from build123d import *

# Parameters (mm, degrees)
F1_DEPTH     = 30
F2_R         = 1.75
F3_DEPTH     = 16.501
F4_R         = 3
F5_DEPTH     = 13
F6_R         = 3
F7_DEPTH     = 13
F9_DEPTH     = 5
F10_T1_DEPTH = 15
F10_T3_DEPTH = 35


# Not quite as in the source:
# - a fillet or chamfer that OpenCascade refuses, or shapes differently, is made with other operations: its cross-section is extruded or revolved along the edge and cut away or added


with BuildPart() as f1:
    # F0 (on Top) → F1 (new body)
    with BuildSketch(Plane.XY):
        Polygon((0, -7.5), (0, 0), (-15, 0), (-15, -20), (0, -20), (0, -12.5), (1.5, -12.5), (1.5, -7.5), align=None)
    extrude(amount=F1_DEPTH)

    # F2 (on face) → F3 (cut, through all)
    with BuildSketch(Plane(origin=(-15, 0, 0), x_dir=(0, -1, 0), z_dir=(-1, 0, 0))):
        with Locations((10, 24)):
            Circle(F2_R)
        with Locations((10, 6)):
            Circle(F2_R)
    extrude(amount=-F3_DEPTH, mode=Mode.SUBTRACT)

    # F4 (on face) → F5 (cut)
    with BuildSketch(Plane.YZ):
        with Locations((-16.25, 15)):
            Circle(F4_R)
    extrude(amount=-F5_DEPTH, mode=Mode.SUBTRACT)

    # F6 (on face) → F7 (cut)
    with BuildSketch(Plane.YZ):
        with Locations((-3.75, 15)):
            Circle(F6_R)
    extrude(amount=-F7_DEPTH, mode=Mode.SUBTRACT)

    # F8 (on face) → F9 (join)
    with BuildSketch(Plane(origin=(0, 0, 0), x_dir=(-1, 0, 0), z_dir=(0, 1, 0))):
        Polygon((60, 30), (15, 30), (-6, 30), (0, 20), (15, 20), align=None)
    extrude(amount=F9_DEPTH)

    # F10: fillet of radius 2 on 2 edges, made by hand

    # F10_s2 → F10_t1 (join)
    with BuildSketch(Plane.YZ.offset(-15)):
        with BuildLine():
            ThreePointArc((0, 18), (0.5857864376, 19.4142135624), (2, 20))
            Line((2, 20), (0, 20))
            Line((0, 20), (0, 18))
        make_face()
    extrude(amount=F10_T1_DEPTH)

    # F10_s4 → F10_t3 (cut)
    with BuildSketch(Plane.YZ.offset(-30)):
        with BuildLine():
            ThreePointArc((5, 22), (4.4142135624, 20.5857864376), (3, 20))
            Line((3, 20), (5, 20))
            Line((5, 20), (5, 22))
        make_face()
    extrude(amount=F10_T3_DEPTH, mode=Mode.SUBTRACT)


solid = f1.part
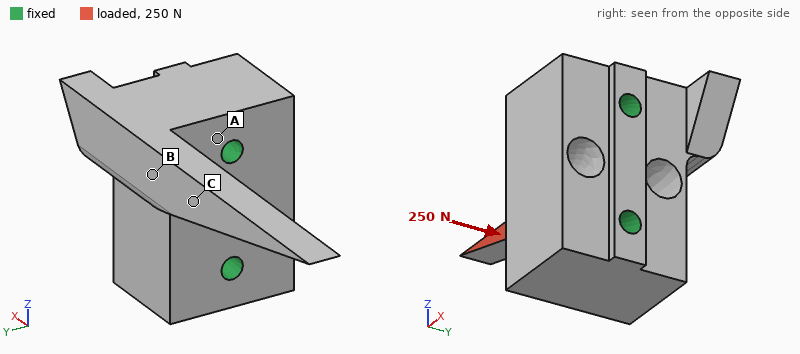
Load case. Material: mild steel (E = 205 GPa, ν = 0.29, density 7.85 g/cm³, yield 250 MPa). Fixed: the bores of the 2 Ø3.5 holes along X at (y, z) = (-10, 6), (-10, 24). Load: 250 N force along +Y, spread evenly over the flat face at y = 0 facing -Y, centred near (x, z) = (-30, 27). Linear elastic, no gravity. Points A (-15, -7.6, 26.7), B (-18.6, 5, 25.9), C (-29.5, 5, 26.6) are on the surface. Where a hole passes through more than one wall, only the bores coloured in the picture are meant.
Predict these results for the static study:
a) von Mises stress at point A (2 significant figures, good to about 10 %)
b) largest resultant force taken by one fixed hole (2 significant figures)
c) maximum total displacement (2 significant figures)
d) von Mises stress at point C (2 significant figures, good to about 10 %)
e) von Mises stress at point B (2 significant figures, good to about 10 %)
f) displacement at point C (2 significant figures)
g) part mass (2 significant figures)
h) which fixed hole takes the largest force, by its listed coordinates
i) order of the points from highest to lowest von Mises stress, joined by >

12 MPa
260 N
0.12 mm
43 MPa
78 MPa
0.027 mm
80 g
(-10, 24)
B > C > A
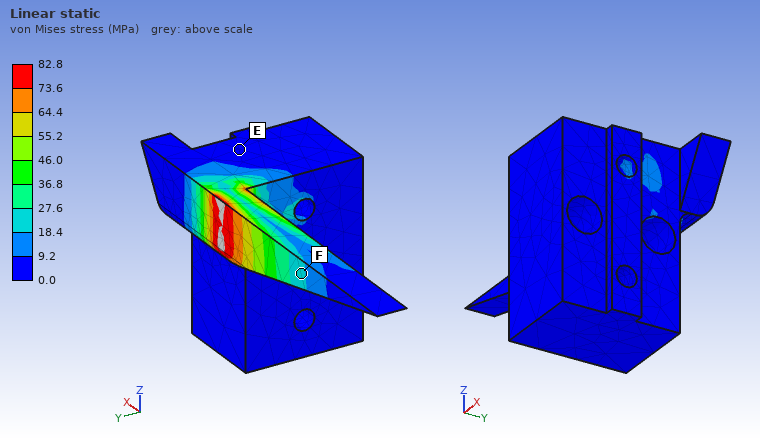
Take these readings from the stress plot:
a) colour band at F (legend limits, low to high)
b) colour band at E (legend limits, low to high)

18.4 to 27.6 MPa
0.0 to 9.2 MPa
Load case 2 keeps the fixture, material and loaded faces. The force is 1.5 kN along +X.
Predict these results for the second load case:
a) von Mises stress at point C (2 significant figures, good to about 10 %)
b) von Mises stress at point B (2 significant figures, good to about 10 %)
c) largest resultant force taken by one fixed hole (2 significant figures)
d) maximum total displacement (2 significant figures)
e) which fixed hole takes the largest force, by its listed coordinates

43 MPa
53 MPa
1.5 kN
0.14 mm
(-10, 24)
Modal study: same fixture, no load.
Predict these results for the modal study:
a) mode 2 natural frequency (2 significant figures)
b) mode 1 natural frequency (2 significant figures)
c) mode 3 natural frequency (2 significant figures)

5100 Hz
3500 Hz
14 kHz
